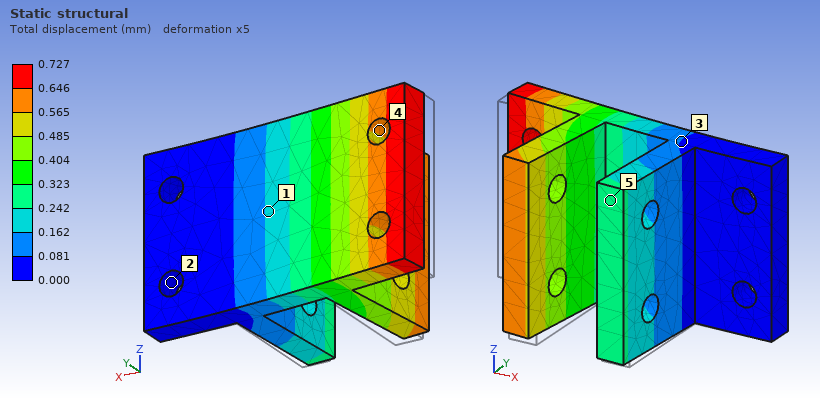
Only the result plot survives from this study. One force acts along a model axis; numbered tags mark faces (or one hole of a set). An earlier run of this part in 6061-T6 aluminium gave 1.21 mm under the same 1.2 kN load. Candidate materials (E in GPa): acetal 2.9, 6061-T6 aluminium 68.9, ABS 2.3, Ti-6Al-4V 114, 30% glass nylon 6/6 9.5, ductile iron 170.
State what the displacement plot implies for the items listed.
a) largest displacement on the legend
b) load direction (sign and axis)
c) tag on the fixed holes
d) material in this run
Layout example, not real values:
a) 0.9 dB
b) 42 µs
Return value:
a) 0.727 mm
b) +Y
c) 2
d) Ti-6Al-4V
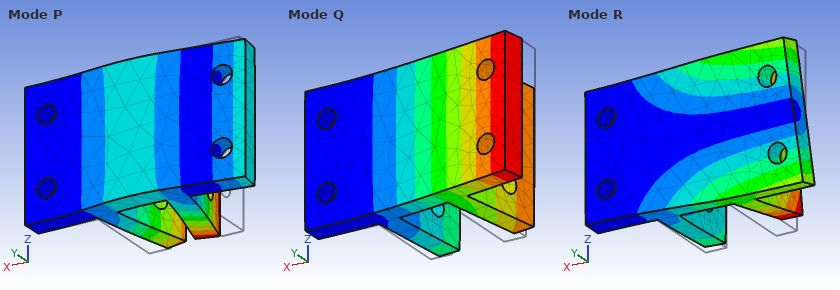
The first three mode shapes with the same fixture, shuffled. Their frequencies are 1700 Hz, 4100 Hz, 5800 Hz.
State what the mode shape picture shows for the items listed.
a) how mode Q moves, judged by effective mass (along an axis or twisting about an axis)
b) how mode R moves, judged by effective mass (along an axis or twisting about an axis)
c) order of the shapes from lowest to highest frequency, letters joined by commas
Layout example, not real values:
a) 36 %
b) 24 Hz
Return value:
a) along Y
b) along Z
c) Q, R, P
